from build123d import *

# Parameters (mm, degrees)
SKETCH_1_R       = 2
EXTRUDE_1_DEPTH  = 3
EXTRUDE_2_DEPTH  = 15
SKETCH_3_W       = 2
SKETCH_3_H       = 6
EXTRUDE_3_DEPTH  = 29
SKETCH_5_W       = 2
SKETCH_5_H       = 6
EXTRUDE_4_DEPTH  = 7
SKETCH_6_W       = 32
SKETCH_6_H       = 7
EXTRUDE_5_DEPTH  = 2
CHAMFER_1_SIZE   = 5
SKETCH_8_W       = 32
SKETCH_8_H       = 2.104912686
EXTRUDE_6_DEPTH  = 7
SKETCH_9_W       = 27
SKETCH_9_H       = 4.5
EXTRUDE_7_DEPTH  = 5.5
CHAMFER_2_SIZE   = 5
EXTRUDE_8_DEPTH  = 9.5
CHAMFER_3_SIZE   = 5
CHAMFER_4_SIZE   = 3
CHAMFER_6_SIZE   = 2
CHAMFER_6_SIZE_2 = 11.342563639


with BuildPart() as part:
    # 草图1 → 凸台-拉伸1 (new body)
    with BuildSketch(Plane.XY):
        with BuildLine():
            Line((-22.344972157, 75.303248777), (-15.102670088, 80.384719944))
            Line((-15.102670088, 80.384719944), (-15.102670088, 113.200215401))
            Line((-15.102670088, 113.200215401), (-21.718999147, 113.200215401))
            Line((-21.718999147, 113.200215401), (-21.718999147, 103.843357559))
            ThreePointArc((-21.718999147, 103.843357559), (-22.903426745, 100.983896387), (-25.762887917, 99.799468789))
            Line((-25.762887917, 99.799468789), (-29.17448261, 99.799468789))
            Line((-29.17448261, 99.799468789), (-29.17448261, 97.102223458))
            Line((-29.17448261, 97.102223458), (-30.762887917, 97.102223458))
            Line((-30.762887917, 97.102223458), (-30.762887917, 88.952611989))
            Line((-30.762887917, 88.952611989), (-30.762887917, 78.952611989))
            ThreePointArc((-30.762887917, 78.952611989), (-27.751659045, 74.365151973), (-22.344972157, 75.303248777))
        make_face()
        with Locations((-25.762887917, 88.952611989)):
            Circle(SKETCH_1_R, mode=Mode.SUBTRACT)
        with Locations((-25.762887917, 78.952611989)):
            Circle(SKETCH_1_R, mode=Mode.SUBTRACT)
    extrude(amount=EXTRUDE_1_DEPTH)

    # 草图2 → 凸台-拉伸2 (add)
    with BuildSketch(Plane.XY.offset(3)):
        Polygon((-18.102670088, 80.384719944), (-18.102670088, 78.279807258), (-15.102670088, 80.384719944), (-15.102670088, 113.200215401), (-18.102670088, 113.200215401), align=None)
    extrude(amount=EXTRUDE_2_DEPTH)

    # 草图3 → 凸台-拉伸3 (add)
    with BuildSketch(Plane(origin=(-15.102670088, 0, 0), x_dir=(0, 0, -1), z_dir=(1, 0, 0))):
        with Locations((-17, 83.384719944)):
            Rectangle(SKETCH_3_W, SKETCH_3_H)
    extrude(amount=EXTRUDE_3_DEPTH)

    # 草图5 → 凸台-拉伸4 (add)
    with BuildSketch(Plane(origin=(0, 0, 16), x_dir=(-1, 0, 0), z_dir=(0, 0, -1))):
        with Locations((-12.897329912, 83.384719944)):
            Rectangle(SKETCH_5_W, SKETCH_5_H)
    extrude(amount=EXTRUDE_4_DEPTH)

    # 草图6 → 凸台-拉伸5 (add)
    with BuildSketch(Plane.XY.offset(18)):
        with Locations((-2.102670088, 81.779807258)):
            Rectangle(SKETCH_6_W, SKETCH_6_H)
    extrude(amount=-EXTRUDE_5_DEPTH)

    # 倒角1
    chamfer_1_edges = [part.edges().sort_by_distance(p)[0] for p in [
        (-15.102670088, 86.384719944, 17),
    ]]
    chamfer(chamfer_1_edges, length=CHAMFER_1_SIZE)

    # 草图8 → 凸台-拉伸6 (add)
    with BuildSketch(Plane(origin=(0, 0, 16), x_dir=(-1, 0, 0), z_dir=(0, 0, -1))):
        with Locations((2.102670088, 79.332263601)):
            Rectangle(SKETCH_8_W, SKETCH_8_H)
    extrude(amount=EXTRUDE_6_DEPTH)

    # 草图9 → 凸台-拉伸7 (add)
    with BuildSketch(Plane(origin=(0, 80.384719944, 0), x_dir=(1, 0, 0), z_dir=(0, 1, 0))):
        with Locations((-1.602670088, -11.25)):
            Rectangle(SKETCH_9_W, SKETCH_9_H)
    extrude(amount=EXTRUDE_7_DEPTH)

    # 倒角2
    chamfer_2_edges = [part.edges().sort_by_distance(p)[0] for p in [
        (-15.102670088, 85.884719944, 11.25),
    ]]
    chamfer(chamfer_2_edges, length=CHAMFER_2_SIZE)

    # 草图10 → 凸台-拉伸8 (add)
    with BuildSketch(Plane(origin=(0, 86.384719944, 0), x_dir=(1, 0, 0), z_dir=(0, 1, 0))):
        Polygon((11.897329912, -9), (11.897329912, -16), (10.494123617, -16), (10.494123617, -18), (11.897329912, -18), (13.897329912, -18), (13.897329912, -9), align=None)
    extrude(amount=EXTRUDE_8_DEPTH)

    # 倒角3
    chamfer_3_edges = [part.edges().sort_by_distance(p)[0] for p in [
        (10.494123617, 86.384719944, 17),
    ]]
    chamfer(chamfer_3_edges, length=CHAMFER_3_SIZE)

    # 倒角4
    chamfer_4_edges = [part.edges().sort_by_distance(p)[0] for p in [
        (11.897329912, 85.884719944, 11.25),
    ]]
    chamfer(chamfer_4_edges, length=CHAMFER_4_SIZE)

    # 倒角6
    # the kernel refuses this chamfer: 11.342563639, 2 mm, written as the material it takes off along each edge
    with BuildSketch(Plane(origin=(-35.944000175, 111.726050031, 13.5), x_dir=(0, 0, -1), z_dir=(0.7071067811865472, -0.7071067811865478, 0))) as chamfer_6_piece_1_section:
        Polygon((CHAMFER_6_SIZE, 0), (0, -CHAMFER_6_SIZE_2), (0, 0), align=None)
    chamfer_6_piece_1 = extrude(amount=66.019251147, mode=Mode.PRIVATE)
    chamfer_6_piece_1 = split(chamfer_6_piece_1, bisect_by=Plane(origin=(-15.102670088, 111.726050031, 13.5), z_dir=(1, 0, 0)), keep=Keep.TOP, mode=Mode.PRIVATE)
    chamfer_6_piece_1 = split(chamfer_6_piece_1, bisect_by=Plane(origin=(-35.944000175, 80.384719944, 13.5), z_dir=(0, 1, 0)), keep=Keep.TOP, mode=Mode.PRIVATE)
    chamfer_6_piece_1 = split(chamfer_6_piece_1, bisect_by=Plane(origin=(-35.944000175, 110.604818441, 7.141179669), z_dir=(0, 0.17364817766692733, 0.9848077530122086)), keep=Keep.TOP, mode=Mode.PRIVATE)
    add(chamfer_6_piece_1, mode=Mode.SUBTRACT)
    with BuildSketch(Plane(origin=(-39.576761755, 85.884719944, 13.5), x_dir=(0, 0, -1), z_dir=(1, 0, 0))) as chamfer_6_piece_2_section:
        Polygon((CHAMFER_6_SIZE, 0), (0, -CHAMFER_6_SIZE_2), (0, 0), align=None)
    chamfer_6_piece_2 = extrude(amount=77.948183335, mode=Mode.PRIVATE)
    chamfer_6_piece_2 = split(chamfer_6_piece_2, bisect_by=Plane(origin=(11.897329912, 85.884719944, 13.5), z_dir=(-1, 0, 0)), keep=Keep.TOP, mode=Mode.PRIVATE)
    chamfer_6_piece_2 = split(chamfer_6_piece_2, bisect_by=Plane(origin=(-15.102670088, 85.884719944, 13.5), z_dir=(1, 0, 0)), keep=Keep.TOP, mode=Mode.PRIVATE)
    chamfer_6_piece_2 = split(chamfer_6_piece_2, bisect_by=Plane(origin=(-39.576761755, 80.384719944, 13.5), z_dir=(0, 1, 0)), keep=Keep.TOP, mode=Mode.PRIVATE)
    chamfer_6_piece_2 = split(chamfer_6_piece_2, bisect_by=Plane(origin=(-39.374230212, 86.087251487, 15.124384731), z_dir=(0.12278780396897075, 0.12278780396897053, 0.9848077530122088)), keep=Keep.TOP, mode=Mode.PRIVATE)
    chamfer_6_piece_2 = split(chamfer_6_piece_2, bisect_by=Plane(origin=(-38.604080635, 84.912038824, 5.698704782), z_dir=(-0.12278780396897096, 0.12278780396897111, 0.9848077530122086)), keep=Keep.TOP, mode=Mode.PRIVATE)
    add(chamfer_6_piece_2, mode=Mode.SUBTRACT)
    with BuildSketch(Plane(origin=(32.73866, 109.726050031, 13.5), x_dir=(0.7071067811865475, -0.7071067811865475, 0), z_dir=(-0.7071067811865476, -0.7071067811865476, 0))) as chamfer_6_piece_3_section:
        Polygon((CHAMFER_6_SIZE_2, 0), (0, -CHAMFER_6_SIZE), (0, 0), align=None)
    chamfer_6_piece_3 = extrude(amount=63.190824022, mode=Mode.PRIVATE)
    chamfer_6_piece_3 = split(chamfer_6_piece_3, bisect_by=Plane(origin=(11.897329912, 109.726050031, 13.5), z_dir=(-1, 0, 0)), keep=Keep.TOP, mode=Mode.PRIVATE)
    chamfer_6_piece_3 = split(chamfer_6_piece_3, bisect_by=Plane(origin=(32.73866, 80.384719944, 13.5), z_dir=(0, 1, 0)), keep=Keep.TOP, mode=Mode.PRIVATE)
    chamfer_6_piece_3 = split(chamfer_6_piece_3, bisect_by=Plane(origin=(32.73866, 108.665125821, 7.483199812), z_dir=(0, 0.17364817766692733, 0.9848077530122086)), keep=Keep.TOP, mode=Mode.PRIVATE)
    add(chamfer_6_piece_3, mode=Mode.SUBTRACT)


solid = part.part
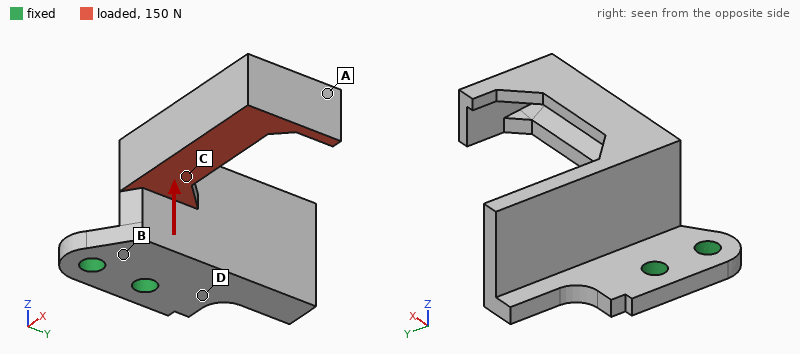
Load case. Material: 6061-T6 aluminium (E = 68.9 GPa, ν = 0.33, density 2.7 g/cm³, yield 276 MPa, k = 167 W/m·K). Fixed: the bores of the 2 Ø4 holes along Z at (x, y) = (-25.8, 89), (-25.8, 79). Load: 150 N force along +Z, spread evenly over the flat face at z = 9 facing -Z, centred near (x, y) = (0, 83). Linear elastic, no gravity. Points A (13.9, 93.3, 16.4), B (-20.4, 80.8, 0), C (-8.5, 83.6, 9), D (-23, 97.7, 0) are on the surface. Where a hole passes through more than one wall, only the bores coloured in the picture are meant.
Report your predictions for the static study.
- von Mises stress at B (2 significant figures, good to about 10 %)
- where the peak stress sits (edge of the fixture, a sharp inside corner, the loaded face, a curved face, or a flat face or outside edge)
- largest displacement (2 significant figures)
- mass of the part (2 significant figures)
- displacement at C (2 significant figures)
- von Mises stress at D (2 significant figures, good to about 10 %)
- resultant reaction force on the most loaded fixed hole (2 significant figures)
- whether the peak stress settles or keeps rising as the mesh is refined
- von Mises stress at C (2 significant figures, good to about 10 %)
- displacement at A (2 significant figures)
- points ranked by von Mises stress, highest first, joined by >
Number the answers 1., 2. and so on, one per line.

1. 84 MPa
2. edge of the fixture
3. 0.56 mm
4. 12 g
5. 0.16 mm
6. 59 MPa
7. 77 N
8. keeps rising
9. 33 MPa
10. 0.55 mm
11. B > D > C > A
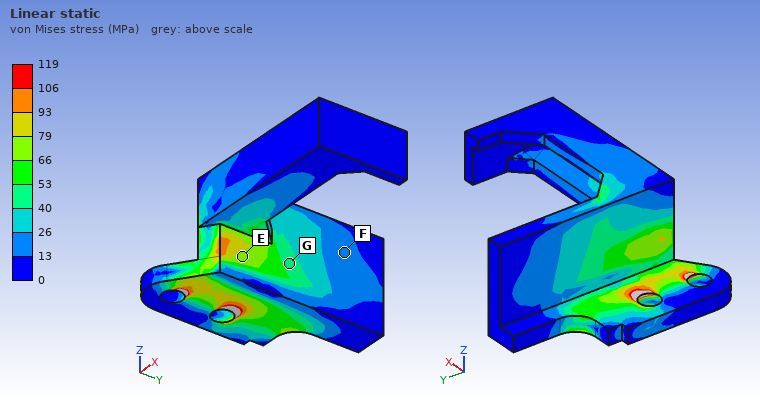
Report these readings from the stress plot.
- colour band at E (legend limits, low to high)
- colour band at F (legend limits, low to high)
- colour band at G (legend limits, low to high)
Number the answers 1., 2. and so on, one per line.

1. 66 to 79 MPa
2. 13 to 26 MPa
3. 40 to 53 MPa
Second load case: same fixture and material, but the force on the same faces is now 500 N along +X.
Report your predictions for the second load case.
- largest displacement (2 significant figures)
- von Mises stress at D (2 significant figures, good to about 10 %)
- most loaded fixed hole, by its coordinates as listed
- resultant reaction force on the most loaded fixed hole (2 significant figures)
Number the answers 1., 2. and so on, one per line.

1. 0.41 mm
2. 61 MPa
3. (-25.8, 79)
4. 290 N
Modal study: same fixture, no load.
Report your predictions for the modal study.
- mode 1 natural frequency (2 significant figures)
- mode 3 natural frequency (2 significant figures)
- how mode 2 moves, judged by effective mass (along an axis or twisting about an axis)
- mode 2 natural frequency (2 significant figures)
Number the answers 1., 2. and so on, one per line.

1. 1300 Hz
2. 4000 Hz
3. along Y
4. 2600 Hz
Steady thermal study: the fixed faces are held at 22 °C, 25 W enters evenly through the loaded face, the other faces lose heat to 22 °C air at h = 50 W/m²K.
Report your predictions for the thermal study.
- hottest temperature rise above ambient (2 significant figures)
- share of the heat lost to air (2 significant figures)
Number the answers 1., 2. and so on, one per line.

1. 75 K
2. 24 %
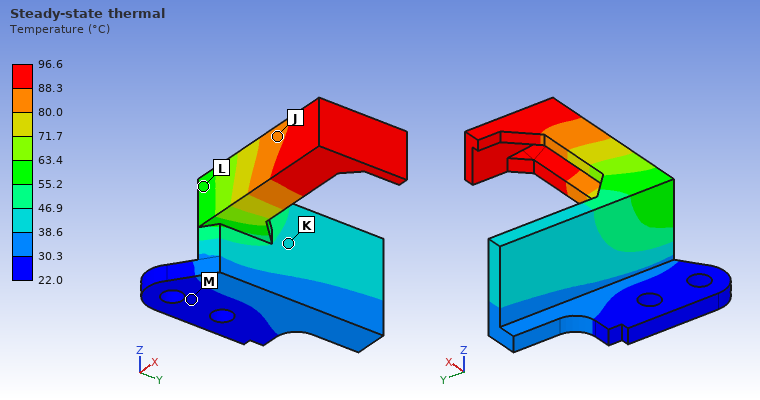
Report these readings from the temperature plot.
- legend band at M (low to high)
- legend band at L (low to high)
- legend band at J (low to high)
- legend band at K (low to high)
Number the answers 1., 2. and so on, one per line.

1. 22.0 to 30.3 °C
2. 55.2 to 63.4 °C
3. 80.0 to 88.3 °C
4. 38.6 to 46.9 °C
